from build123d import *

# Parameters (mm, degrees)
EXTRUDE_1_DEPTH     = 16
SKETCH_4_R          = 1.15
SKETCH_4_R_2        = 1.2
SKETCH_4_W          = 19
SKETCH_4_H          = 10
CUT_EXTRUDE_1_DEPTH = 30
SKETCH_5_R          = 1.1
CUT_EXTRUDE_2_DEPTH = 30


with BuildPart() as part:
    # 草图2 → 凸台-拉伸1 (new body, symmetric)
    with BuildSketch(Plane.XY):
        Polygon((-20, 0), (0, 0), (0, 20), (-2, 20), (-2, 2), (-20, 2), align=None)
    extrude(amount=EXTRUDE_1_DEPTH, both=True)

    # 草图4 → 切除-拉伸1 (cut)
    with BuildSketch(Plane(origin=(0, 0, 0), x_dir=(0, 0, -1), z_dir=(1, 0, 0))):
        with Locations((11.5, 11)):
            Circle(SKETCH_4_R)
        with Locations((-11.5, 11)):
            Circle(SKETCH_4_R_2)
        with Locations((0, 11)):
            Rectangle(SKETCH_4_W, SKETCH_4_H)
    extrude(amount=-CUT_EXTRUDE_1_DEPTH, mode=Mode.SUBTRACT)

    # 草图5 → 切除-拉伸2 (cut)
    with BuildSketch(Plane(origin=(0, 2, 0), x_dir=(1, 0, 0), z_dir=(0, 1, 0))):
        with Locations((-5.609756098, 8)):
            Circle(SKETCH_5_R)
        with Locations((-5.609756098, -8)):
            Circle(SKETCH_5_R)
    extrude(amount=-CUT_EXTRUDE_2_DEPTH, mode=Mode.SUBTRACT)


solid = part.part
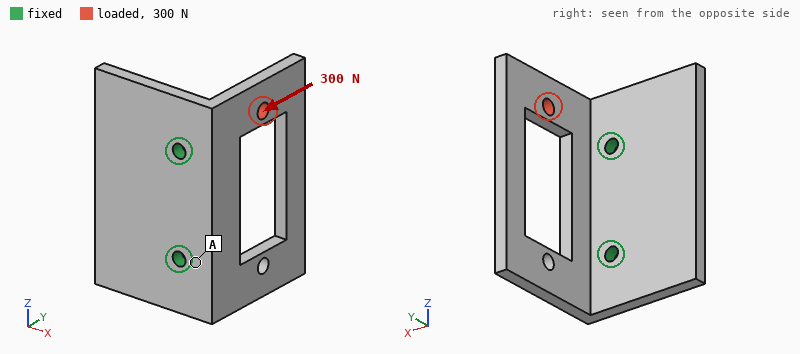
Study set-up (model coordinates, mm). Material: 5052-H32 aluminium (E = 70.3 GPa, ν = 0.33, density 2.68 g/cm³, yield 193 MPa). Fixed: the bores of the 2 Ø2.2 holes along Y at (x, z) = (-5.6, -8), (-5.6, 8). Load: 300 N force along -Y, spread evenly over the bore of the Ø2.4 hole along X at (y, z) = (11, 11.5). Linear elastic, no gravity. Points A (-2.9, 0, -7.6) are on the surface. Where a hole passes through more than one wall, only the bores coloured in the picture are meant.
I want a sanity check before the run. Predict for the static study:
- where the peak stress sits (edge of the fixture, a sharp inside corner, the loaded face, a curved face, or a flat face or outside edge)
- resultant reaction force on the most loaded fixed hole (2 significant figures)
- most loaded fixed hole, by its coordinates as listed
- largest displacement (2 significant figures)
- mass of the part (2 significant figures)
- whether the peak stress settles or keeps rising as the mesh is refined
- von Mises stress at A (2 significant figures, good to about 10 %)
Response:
edge of the fixture
340 N
(-5.6, 8)
98 µm
5.4 g
keeps rising
18 MPa
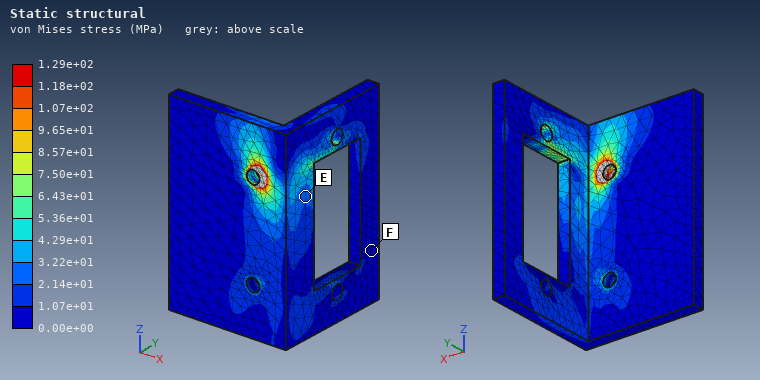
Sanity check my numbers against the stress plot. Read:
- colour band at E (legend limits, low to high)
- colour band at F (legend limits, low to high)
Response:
2.14e+01 to 3.22e+01 MPa
0.00e+00 to 1.07e+01 MPa
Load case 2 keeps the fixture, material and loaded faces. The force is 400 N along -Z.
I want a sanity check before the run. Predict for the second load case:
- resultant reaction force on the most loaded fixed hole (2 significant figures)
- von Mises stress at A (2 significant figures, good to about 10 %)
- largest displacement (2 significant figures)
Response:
300 N
53 MPa
94 µm
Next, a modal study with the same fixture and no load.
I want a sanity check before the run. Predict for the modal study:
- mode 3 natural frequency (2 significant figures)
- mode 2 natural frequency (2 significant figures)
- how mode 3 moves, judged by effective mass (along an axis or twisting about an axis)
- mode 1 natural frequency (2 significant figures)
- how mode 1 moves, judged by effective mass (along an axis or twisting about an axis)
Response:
7400 Hz
5200 Hz
along Y
2900 Hz
along X
